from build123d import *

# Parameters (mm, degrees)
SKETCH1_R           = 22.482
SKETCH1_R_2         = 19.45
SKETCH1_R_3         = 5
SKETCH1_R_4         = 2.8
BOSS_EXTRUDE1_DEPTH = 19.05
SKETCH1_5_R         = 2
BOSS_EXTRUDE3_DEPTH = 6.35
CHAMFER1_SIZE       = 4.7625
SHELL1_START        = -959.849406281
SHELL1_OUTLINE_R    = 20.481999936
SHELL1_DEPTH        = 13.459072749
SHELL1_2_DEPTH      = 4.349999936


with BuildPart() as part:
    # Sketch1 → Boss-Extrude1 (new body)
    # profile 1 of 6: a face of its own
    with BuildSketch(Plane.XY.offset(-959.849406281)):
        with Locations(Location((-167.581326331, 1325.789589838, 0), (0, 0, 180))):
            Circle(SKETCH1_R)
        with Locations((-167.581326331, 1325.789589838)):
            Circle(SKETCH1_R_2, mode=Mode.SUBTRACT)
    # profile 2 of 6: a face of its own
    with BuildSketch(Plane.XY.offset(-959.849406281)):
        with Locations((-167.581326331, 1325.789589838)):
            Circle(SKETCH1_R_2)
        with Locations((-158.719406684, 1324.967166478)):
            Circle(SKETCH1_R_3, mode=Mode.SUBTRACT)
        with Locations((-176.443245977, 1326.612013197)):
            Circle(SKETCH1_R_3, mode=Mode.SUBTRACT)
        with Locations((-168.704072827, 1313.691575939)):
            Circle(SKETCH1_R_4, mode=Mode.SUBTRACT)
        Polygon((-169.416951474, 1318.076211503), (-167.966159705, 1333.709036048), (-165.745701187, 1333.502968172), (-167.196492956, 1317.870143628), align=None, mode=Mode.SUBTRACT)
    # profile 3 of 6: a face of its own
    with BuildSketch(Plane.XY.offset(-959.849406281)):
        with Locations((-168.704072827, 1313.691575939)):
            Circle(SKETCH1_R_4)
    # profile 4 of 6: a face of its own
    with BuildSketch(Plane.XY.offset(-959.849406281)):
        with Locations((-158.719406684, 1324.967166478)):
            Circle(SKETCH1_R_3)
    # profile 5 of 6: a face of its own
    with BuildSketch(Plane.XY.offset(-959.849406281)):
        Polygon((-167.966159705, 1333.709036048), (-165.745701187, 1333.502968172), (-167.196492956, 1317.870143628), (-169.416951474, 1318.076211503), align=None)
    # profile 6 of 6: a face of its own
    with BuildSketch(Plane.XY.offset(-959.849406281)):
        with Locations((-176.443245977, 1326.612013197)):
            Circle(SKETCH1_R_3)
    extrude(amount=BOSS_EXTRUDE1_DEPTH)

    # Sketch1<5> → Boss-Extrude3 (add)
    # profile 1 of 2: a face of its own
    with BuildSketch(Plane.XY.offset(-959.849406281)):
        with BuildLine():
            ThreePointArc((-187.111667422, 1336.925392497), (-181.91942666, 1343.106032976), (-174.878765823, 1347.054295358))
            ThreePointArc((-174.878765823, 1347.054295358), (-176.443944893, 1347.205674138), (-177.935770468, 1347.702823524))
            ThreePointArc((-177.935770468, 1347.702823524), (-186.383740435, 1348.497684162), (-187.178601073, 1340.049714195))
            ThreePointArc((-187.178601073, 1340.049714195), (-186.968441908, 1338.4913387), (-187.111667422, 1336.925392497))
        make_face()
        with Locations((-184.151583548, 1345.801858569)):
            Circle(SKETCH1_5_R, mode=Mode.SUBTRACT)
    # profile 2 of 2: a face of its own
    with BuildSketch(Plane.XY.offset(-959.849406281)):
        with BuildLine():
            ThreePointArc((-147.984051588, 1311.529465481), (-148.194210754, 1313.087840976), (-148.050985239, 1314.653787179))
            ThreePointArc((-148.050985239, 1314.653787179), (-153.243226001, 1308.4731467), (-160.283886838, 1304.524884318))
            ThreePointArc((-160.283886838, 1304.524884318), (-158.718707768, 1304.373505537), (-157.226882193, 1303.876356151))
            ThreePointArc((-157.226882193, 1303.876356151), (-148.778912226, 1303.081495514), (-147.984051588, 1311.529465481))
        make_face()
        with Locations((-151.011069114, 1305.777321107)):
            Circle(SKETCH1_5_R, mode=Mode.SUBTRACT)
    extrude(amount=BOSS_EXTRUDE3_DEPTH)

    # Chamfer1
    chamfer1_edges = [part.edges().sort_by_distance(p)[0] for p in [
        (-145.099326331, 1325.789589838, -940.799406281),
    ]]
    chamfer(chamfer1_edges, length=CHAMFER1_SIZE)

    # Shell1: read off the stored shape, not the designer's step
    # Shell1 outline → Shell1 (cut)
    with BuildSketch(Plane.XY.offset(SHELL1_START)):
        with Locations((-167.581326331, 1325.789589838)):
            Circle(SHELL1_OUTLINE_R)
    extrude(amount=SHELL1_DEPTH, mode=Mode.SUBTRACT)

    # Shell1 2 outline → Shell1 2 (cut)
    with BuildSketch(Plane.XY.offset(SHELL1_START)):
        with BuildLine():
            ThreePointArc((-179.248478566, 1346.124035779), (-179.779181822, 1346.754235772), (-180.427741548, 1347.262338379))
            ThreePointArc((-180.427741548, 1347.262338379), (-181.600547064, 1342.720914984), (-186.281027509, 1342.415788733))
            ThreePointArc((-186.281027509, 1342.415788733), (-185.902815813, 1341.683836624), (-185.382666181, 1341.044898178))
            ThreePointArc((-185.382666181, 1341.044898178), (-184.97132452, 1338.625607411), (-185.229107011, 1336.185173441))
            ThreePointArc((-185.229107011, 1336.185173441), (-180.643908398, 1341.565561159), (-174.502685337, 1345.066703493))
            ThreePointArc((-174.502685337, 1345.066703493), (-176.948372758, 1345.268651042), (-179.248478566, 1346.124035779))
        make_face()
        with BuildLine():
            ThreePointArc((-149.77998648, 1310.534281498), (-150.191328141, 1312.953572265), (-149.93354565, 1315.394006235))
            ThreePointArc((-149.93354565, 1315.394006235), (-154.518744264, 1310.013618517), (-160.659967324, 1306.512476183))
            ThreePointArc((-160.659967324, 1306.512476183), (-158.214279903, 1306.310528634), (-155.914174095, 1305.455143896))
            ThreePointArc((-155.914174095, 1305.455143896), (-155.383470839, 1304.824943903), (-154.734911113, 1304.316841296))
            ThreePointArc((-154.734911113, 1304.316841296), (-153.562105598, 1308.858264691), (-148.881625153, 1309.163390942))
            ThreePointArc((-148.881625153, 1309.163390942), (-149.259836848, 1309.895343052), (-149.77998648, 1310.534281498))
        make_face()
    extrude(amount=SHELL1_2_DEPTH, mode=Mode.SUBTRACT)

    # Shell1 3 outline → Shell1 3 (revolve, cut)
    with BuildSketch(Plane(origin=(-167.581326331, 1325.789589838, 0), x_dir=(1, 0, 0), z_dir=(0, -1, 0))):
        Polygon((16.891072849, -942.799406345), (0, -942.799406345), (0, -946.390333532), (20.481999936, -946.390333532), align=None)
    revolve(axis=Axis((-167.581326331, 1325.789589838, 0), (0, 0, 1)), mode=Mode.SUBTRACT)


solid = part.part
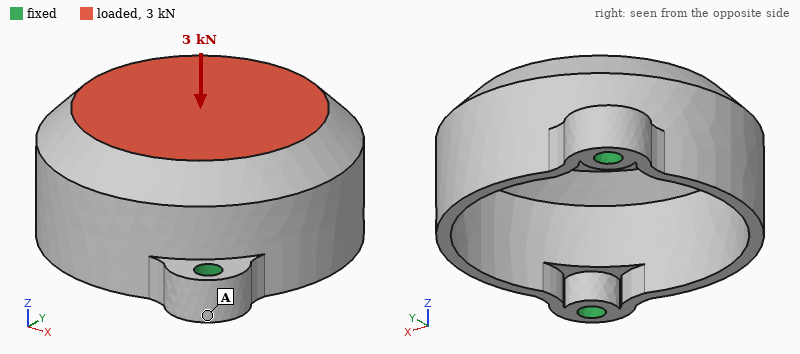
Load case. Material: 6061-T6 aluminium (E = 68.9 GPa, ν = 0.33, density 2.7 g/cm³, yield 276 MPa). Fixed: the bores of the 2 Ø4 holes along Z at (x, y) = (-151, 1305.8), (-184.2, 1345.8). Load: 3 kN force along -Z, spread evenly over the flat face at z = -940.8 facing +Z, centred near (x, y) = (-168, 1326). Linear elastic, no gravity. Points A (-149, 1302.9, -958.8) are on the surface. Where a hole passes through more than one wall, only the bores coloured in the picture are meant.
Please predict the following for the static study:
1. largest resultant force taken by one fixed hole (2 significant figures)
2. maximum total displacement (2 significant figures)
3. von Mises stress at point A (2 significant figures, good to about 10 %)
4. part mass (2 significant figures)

1.7 kN
0.19 mm
24 MPa
21 g
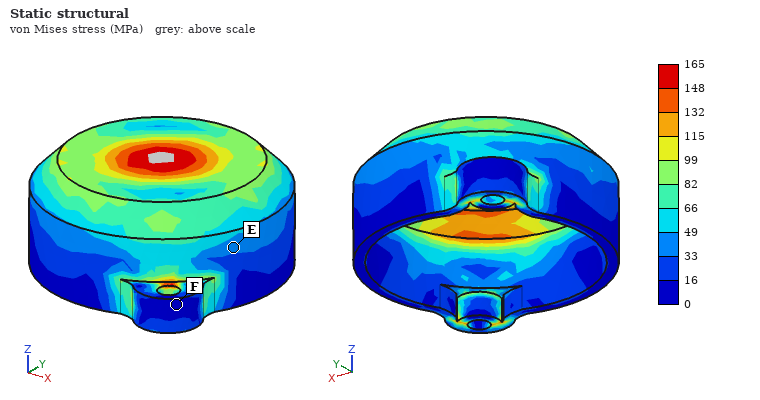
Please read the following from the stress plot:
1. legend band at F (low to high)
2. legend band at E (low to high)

0 to 16 MPa
33 to 49 MPa
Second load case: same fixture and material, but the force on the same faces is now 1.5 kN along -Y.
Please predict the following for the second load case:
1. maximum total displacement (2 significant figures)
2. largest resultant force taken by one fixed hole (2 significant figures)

0.10 mm
830 N
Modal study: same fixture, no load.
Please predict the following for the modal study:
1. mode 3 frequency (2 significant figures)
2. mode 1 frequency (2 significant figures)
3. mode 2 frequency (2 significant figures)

7200 Hz
4200 Hz
6500 Hz
